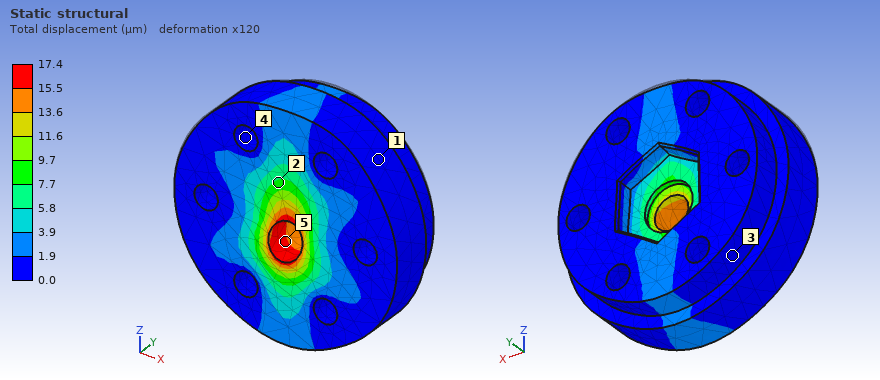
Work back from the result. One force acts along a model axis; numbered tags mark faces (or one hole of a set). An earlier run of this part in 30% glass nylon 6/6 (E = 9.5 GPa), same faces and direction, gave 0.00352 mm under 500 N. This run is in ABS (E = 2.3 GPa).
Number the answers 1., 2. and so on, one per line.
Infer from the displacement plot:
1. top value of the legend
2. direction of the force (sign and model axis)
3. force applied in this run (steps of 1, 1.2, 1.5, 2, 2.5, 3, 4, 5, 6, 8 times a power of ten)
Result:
1. 17.4 µm
2. -Z
3. 600 N
